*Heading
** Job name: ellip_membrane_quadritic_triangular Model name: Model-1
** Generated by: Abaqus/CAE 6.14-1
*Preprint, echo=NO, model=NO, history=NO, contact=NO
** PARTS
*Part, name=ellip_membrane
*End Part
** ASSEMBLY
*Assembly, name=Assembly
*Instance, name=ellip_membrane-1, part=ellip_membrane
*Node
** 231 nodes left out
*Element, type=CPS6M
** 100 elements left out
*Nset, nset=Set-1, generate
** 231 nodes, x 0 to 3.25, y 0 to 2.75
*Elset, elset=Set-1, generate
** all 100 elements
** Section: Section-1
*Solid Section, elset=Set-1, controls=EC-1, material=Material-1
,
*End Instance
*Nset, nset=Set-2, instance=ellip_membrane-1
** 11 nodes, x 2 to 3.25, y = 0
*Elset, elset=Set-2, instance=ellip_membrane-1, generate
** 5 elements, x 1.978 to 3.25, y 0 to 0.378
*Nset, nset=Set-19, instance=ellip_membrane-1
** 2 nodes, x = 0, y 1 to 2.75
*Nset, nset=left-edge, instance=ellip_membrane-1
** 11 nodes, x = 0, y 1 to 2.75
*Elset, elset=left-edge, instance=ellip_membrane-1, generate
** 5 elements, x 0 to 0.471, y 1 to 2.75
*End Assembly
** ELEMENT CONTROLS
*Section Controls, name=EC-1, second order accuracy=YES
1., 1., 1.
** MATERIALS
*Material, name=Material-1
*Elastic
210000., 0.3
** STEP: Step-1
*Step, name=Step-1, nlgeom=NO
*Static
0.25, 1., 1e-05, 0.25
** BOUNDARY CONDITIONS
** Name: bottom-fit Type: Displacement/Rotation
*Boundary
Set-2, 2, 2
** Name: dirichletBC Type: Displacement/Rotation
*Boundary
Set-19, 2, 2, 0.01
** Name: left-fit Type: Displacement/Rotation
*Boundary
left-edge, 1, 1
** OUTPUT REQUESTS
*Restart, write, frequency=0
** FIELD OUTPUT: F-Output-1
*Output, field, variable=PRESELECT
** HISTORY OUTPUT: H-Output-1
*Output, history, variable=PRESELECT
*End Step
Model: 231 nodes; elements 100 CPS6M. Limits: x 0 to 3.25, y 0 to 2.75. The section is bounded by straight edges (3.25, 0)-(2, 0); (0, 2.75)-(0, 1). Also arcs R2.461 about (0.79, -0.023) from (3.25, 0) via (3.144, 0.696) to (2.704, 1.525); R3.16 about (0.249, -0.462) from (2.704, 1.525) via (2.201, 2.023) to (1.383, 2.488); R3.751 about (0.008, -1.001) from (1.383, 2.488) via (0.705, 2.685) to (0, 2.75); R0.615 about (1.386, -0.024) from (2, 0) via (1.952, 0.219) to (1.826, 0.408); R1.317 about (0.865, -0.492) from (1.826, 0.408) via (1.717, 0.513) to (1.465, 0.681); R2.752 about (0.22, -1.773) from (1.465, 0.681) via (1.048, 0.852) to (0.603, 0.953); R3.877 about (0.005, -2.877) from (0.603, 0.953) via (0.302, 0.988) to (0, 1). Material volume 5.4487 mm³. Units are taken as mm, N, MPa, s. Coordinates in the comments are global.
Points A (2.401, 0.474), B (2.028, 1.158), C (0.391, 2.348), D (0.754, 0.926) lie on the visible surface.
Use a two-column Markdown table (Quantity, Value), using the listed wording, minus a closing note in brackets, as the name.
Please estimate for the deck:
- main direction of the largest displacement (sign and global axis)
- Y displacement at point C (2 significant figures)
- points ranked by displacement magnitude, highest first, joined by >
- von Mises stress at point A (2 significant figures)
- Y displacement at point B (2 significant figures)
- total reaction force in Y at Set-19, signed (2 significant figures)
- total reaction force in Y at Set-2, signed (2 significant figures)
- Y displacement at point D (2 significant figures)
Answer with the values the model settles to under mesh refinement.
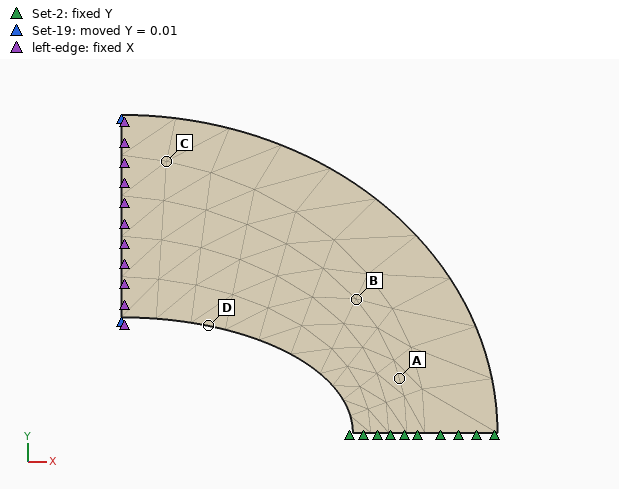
| Quantity | Value |
|---|---|
| main direction of the largest displacement | +Y |
| Y displacement at point C | 0.0083 mm |
| points ranked by displacement magnitude, highest first, joined by > | C > D > A > B |
| von Mises stress at point A | 190 MPa |
| Y displacement at point B | 0.0021 mm |
| total reaction force in Y at Set-19, signed | 160 N |
| total reaction force in Y at Set-2, signed | -160 N |
| Y displacement at point D | 0.0071 mm |
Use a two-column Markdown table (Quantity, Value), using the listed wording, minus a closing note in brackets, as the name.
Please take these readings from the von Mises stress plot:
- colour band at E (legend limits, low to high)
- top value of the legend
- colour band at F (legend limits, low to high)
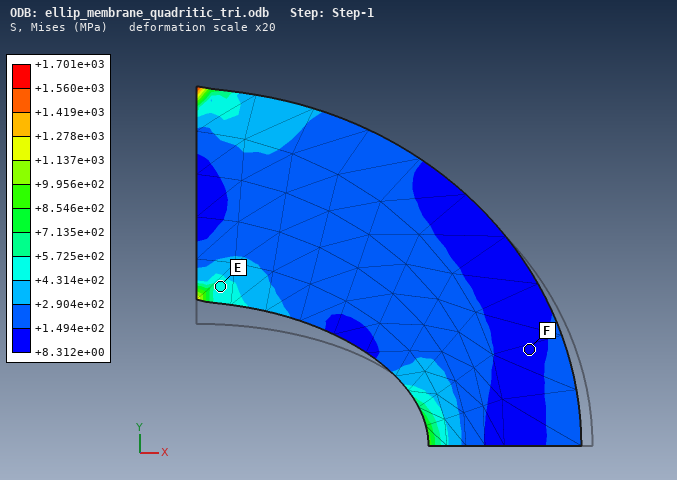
| Quantity | Value |
|---|---|
| colour band at E | +4.314e+02 to +5.725e+02 MPa |
| top value of the legend | +1.701e+03 MPa |
| colour band at F | +8.312e+00 to +1.494e+02 MPa |
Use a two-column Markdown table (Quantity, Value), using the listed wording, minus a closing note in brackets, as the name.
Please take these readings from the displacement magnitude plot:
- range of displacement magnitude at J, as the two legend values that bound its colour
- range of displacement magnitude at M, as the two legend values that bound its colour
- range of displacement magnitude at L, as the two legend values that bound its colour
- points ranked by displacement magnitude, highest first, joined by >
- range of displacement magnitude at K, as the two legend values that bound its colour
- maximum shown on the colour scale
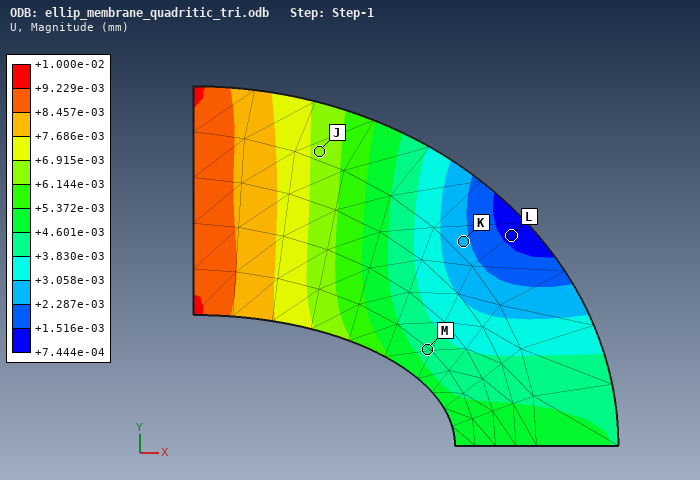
| Quantity | Value |
|---|---|
| range of displacement magnitude at J, as the two legend values that bound its colour | +6.144e-03 to +6.915e-03 mm |
| range of displacement magnitude at M, as the two legend values that bound its colour | +3.830e-03 to +4.601e-03 mm |
| range of displacement magnitude at L, as the two legend values that bound its colour | +7.444e-04 to +1.516e-03 mm |
| points ranked by displacement magnitude, highest first, joined by > | J > M > K > L |
| range of displacement magnitude at K, as the two legend values that bound its colour | +2.287e-03 to +3.058e-03 mm |
| maximum shown on the colour scale | +1.000e-02 mm |
